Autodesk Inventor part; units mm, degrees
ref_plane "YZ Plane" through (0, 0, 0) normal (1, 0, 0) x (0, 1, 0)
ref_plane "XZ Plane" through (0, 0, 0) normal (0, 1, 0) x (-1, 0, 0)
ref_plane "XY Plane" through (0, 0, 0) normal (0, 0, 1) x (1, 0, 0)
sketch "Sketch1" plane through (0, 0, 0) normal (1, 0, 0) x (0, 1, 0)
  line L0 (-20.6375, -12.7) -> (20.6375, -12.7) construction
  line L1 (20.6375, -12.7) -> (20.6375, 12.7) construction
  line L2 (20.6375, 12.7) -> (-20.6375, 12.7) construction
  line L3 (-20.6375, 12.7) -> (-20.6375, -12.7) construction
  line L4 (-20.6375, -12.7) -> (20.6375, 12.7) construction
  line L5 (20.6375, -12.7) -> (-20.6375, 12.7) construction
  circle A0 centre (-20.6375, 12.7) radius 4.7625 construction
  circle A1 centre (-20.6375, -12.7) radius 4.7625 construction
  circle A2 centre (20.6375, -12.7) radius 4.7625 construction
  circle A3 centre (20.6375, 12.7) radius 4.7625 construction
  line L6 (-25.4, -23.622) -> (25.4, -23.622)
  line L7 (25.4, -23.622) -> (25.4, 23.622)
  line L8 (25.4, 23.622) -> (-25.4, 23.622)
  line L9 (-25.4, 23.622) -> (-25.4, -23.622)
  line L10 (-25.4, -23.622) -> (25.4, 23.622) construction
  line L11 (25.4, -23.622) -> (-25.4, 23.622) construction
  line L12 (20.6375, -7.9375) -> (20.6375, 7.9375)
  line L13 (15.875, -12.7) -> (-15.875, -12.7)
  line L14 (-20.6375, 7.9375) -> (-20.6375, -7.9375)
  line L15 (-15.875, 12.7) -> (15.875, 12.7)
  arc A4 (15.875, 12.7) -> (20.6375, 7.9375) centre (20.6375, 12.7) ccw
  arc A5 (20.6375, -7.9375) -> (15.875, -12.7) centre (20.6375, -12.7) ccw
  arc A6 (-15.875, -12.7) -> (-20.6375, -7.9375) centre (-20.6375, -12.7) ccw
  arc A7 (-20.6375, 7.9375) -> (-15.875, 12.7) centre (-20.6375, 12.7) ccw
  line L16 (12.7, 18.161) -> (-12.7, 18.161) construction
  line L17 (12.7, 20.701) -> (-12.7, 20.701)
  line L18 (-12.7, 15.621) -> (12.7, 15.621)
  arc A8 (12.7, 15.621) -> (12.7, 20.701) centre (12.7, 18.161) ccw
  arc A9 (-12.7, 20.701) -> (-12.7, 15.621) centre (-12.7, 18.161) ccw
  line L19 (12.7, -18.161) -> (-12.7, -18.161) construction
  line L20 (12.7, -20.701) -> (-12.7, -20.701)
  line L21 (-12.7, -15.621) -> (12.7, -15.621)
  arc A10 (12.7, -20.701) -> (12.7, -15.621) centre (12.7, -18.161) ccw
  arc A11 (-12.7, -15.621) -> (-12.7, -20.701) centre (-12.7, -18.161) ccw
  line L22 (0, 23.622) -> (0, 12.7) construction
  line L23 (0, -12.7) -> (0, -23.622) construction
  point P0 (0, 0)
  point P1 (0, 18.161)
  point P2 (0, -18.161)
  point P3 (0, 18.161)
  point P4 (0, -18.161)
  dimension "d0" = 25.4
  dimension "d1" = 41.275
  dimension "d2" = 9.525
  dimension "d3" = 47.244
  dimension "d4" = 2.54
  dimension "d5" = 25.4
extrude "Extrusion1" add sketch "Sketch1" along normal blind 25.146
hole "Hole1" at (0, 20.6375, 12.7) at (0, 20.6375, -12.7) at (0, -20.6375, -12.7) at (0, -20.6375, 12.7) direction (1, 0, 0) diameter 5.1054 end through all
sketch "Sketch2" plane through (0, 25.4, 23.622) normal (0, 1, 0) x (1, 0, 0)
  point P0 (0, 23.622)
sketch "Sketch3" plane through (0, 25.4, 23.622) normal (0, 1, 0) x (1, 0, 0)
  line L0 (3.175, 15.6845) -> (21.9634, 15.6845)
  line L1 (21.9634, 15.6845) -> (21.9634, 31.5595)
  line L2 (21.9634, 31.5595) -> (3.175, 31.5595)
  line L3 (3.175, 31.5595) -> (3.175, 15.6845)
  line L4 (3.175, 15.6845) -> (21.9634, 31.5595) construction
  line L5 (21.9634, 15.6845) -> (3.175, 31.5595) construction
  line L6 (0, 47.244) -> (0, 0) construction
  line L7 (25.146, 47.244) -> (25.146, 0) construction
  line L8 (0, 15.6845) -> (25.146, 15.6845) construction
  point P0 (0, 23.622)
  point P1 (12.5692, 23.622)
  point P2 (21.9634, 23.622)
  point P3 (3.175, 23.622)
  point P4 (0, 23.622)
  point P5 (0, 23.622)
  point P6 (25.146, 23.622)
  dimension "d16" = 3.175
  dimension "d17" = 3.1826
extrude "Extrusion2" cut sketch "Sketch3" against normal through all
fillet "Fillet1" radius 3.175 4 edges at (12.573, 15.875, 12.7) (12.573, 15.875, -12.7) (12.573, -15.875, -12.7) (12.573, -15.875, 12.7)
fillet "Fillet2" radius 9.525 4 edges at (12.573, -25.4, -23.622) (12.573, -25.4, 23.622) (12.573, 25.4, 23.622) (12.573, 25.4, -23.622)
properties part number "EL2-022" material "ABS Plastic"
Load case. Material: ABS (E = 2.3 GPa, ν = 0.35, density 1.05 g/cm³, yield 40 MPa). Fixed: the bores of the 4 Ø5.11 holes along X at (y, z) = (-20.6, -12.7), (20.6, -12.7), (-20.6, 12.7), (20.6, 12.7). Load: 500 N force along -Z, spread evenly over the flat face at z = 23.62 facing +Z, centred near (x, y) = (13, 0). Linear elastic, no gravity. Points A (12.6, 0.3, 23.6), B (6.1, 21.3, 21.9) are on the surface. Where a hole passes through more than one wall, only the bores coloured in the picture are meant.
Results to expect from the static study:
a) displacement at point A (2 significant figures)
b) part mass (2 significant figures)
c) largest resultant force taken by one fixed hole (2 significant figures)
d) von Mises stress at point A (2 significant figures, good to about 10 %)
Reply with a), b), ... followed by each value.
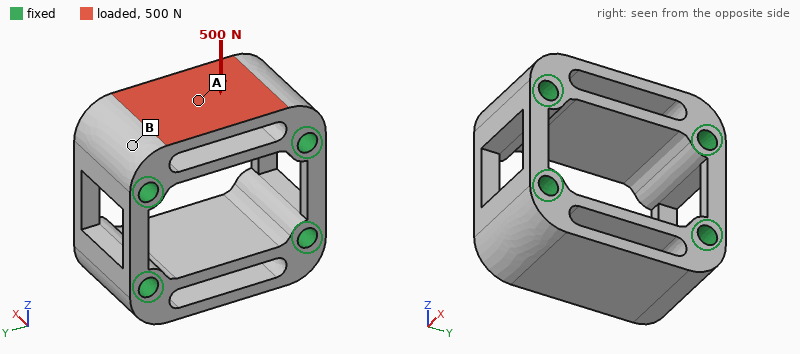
a) 0.33 mm
b) 23 g
c) 320 N
d) 18 MPa
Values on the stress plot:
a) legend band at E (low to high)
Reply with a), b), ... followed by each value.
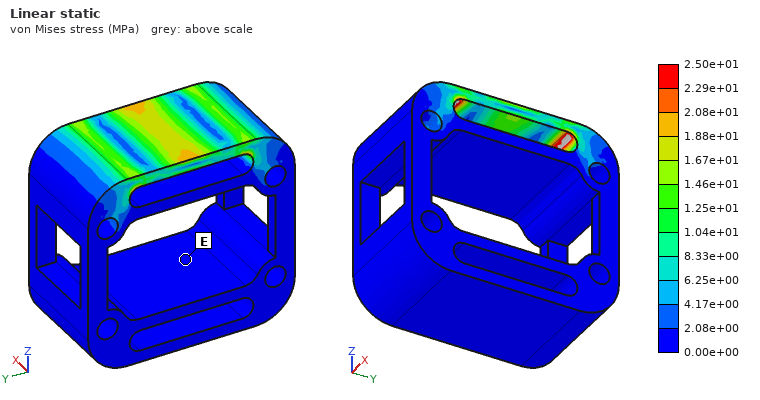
a) 0.00e+00 to 2.08e+00 MPa
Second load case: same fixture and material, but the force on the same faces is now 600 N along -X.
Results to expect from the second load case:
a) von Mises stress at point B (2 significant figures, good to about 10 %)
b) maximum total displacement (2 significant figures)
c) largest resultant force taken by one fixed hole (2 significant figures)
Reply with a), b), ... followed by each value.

a) 1.4 MPa
b) 0.13 mm
c) 300 N
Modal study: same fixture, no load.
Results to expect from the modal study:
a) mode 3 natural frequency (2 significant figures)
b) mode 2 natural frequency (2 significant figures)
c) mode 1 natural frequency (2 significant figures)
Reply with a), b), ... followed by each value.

a) 4700 Hz
b) 4400 Hz
c) 4400 Hz
